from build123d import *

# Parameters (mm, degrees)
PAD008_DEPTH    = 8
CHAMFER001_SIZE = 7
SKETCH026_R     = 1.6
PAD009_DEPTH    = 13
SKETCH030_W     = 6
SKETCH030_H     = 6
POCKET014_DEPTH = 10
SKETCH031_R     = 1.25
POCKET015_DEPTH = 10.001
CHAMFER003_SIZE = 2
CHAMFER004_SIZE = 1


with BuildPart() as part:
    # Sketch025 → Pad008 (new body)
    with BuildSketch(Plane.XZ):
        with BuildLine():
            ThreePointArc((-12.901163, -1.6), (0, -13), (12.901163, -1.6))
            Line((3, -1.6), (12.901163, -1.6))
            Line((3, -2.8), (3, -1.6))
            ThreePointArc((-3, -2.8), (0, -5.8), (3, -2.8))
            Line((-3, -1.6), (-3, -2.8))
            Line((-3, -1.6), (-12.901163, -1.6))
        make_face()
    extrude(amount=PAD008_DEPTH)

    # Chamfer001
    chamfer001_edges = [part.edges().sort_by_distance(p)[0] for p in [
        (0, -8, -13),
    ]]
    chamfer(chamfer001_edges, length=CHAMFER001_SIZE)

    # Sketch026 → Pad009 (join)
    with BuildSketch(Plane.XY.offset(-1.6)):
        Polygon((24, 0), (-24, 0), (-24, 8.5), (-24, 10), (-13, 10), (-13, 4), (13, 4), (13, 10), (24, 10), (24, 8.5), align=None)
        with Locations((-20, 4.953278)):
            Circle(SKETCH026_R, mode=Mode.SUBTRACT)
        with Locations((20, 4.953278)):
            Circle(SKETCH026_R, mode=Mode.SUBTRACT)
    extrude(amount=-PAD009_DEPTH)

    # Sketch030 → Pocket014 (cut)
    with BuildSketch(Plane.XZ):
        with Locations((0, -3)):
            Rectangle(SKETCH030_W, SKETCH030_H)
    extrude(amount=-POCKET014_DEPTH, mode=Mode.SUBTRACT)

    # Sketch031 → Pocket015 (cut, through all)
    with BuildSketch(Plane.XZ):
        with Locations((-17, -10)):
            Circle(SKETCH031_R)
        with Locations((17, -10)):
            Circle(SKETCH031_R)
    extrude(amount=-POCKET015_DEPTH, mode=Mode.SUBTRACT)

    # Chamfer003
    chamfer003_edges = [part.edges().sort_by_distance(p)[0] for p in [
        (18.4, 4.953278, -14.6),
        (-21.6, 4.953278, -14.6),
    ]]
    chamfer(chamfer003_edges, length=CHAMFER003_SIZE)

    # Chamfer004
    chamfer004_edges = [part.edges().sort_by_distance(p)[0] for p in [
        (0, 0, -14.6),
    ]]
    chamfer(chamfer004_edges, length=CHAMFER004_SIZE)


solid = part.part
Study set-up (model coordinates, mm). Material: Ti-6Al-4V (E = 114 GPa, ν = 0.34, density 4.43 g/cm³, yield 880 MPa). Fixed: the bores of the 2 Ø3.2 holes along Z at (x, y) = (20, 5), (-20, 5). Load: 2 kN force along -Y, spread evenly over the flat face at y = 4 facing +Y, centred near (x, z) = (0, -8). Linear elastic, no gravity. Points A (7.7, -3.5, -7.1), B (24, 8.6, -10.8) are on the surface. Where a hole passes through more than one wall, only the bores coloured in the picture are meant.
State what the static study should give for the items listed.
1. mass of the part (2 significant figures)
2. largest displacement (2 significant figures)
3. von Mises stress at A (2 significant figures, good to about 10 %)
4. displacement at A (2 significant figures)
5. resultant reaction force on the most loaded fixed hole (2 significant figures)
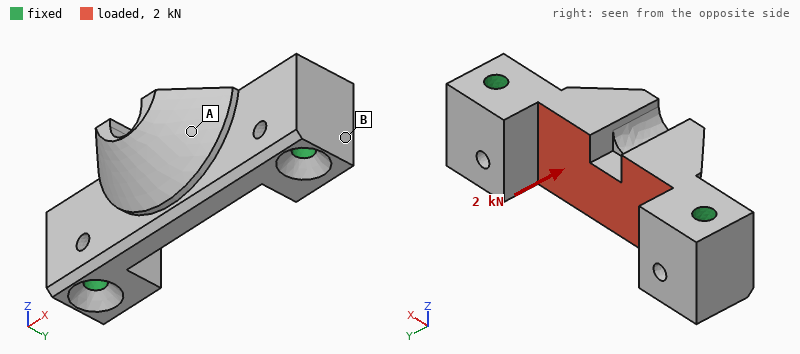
20 g
19 µm
41 MPa
11 µm
1.3 kN
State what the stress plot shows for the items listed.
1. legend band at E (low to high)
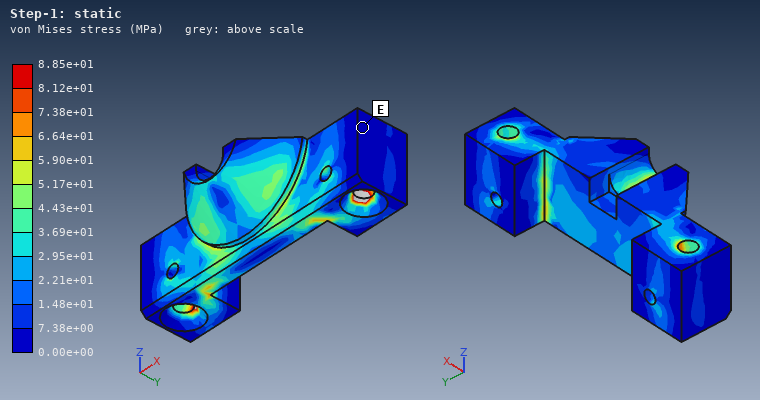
0.00e+00 to 7.38e+00 MPa
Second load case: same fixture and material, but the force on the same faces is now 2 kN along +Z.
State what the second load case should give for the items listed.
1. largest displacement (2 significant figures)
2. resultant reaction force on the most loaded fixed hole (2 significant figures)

16 µm
1.0 kN
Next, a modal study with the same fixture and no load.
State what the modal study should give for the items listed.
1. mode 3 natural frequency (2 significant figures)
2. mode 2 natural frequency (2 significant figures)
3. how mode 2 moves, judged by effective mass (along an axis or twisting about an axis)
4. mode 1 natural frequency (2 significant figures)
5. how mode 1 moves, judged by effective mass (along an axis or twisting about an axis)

30 kHz
22 kHz
along Y
19 kHz
along Z
